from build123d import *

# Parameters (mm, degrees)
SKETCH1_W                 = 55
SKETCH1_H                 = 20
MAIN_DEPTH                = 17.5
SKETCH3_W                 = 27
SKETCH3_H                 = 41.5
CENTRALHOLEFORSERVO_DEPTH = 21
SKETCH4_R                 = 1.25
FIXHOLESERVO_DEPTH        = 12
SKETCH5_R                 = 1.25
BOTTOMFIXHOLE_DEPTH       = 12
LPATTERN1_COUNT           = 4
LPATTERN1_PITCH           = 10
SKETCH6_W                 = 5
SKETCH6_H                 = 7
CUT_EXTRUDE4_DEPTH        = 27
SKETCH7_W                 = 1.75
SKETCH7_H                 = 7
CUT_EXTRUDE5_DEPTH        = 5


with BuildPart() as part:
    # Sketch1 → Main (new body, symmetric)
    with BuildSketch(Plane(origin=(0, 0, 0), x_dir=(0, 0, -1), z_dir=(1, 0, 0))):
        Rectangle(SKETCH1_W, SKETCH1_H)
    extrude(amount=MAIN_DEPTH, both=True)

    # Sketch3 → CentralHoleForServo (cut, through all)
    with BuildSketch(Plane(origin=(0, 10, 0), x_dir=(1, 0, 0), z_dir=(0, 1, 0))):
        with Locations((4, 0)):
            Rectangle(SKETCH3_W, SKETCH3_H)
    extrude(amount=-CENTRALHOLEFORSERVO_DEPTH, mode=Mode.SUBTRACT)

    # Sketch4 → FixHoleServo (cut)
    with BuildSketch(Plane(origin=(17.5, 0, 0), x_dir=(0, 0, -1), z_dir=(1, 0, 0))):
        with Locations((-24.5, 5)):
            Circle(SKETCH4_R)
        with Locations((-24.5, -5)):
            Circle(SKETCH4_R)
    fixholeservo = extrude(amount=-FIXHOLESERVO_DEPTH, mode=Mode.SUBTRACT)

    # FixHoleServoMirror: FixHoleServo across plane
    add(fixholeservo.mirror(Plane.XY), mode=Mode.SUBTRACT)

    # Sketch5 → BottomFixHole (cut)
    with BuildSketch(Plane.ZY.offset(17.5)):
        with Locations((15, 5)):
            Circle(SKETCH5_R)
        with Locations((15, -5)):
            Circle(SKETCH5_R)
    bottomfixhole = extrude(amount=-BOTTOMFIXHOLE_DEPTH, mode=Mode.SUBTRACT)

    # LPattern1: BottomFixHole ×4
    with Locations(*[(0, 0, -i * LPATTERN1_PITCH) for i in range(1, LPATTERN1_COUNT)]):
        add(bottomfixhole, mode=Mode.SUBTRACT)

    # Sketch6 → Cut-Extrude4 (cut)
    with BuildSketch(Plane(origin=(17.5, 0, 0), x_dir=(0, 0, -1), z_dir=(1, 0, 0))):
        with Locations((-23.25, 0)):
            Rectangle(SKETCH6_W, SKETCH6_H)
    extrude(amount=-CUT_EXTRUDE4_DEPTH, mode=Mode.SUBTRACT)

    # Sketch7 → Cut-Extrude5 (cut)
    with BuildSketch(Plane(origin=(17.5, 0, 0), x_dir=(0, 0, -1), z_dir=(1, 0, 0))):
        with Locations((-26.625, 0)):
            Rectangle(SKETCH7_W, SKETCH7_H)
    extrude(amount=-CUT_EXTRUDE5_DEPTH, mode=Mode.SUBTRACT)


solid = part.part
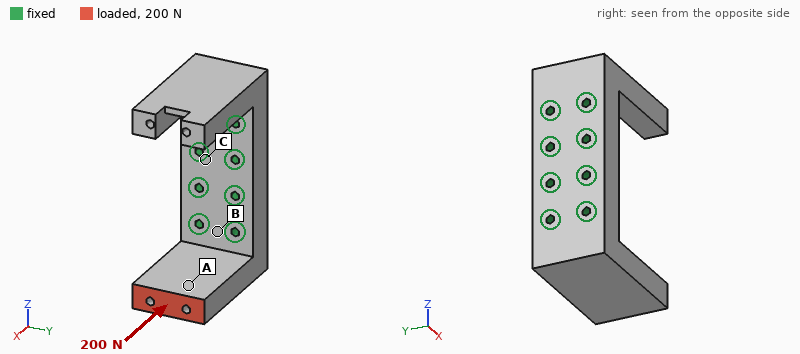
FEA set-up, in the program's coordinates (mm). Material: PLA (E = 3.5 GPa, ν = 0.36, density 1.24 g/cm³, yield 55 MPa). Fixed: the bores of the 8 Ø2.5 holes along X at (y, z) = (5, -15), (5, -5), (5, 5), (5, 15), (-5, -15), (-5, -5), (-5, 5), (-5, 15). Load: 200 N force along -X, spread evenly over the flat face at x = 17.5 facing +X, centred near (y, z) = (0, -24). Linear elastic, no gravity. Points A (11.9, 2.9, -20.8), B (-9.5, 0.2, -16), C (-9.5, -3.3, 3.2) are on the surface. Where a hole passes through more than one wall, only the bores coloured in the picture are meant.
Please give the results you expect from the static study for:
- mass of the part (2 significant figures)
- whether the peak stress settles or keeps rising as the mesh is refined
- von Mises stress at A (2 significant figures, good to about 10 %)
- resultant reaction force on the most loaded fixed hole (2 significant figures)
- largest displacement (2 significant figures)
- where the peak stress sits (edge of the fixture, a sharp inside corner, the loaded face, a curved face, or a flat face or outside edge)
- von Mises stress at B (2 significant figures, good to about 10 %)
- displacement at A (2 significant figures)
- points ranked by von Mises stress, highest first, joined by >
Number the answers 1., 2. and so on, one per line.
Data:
1. 18 g
2. keeps rising
3. 1.6 MPa
4. 110 N
5. 0.12 mm
6. edge of the fixture
7. 4.0 MPa
8. 0.088 mm
9. B > A > C
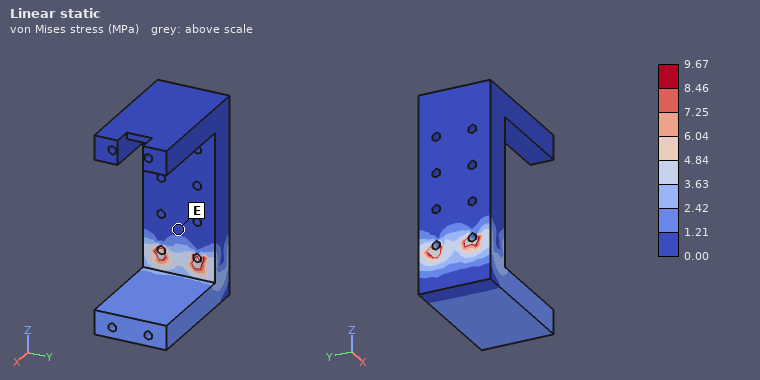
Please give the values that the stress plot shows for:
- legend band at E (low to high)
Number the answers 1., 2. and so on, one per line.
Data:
1. 0.00 to 1.21 MPa
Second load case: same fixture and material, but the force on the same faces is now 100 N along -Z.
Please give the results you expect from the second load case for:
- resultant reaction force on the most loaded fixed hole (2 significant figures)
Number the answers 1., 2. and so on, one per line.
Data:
1. 64 N
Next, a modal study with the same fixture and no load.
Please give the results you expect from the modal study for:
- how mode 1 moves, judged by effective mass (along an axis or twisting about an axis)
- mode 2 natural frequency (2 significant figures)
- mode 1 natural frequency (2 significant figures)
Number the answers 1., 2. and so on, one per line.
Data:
1. along Z
2. 1800 Hz
3. 1600 Hz
